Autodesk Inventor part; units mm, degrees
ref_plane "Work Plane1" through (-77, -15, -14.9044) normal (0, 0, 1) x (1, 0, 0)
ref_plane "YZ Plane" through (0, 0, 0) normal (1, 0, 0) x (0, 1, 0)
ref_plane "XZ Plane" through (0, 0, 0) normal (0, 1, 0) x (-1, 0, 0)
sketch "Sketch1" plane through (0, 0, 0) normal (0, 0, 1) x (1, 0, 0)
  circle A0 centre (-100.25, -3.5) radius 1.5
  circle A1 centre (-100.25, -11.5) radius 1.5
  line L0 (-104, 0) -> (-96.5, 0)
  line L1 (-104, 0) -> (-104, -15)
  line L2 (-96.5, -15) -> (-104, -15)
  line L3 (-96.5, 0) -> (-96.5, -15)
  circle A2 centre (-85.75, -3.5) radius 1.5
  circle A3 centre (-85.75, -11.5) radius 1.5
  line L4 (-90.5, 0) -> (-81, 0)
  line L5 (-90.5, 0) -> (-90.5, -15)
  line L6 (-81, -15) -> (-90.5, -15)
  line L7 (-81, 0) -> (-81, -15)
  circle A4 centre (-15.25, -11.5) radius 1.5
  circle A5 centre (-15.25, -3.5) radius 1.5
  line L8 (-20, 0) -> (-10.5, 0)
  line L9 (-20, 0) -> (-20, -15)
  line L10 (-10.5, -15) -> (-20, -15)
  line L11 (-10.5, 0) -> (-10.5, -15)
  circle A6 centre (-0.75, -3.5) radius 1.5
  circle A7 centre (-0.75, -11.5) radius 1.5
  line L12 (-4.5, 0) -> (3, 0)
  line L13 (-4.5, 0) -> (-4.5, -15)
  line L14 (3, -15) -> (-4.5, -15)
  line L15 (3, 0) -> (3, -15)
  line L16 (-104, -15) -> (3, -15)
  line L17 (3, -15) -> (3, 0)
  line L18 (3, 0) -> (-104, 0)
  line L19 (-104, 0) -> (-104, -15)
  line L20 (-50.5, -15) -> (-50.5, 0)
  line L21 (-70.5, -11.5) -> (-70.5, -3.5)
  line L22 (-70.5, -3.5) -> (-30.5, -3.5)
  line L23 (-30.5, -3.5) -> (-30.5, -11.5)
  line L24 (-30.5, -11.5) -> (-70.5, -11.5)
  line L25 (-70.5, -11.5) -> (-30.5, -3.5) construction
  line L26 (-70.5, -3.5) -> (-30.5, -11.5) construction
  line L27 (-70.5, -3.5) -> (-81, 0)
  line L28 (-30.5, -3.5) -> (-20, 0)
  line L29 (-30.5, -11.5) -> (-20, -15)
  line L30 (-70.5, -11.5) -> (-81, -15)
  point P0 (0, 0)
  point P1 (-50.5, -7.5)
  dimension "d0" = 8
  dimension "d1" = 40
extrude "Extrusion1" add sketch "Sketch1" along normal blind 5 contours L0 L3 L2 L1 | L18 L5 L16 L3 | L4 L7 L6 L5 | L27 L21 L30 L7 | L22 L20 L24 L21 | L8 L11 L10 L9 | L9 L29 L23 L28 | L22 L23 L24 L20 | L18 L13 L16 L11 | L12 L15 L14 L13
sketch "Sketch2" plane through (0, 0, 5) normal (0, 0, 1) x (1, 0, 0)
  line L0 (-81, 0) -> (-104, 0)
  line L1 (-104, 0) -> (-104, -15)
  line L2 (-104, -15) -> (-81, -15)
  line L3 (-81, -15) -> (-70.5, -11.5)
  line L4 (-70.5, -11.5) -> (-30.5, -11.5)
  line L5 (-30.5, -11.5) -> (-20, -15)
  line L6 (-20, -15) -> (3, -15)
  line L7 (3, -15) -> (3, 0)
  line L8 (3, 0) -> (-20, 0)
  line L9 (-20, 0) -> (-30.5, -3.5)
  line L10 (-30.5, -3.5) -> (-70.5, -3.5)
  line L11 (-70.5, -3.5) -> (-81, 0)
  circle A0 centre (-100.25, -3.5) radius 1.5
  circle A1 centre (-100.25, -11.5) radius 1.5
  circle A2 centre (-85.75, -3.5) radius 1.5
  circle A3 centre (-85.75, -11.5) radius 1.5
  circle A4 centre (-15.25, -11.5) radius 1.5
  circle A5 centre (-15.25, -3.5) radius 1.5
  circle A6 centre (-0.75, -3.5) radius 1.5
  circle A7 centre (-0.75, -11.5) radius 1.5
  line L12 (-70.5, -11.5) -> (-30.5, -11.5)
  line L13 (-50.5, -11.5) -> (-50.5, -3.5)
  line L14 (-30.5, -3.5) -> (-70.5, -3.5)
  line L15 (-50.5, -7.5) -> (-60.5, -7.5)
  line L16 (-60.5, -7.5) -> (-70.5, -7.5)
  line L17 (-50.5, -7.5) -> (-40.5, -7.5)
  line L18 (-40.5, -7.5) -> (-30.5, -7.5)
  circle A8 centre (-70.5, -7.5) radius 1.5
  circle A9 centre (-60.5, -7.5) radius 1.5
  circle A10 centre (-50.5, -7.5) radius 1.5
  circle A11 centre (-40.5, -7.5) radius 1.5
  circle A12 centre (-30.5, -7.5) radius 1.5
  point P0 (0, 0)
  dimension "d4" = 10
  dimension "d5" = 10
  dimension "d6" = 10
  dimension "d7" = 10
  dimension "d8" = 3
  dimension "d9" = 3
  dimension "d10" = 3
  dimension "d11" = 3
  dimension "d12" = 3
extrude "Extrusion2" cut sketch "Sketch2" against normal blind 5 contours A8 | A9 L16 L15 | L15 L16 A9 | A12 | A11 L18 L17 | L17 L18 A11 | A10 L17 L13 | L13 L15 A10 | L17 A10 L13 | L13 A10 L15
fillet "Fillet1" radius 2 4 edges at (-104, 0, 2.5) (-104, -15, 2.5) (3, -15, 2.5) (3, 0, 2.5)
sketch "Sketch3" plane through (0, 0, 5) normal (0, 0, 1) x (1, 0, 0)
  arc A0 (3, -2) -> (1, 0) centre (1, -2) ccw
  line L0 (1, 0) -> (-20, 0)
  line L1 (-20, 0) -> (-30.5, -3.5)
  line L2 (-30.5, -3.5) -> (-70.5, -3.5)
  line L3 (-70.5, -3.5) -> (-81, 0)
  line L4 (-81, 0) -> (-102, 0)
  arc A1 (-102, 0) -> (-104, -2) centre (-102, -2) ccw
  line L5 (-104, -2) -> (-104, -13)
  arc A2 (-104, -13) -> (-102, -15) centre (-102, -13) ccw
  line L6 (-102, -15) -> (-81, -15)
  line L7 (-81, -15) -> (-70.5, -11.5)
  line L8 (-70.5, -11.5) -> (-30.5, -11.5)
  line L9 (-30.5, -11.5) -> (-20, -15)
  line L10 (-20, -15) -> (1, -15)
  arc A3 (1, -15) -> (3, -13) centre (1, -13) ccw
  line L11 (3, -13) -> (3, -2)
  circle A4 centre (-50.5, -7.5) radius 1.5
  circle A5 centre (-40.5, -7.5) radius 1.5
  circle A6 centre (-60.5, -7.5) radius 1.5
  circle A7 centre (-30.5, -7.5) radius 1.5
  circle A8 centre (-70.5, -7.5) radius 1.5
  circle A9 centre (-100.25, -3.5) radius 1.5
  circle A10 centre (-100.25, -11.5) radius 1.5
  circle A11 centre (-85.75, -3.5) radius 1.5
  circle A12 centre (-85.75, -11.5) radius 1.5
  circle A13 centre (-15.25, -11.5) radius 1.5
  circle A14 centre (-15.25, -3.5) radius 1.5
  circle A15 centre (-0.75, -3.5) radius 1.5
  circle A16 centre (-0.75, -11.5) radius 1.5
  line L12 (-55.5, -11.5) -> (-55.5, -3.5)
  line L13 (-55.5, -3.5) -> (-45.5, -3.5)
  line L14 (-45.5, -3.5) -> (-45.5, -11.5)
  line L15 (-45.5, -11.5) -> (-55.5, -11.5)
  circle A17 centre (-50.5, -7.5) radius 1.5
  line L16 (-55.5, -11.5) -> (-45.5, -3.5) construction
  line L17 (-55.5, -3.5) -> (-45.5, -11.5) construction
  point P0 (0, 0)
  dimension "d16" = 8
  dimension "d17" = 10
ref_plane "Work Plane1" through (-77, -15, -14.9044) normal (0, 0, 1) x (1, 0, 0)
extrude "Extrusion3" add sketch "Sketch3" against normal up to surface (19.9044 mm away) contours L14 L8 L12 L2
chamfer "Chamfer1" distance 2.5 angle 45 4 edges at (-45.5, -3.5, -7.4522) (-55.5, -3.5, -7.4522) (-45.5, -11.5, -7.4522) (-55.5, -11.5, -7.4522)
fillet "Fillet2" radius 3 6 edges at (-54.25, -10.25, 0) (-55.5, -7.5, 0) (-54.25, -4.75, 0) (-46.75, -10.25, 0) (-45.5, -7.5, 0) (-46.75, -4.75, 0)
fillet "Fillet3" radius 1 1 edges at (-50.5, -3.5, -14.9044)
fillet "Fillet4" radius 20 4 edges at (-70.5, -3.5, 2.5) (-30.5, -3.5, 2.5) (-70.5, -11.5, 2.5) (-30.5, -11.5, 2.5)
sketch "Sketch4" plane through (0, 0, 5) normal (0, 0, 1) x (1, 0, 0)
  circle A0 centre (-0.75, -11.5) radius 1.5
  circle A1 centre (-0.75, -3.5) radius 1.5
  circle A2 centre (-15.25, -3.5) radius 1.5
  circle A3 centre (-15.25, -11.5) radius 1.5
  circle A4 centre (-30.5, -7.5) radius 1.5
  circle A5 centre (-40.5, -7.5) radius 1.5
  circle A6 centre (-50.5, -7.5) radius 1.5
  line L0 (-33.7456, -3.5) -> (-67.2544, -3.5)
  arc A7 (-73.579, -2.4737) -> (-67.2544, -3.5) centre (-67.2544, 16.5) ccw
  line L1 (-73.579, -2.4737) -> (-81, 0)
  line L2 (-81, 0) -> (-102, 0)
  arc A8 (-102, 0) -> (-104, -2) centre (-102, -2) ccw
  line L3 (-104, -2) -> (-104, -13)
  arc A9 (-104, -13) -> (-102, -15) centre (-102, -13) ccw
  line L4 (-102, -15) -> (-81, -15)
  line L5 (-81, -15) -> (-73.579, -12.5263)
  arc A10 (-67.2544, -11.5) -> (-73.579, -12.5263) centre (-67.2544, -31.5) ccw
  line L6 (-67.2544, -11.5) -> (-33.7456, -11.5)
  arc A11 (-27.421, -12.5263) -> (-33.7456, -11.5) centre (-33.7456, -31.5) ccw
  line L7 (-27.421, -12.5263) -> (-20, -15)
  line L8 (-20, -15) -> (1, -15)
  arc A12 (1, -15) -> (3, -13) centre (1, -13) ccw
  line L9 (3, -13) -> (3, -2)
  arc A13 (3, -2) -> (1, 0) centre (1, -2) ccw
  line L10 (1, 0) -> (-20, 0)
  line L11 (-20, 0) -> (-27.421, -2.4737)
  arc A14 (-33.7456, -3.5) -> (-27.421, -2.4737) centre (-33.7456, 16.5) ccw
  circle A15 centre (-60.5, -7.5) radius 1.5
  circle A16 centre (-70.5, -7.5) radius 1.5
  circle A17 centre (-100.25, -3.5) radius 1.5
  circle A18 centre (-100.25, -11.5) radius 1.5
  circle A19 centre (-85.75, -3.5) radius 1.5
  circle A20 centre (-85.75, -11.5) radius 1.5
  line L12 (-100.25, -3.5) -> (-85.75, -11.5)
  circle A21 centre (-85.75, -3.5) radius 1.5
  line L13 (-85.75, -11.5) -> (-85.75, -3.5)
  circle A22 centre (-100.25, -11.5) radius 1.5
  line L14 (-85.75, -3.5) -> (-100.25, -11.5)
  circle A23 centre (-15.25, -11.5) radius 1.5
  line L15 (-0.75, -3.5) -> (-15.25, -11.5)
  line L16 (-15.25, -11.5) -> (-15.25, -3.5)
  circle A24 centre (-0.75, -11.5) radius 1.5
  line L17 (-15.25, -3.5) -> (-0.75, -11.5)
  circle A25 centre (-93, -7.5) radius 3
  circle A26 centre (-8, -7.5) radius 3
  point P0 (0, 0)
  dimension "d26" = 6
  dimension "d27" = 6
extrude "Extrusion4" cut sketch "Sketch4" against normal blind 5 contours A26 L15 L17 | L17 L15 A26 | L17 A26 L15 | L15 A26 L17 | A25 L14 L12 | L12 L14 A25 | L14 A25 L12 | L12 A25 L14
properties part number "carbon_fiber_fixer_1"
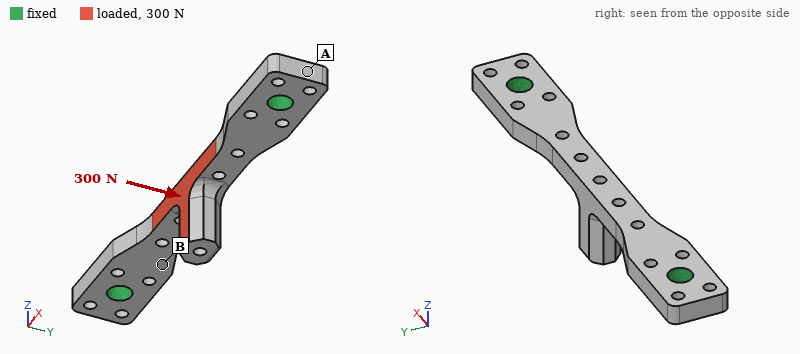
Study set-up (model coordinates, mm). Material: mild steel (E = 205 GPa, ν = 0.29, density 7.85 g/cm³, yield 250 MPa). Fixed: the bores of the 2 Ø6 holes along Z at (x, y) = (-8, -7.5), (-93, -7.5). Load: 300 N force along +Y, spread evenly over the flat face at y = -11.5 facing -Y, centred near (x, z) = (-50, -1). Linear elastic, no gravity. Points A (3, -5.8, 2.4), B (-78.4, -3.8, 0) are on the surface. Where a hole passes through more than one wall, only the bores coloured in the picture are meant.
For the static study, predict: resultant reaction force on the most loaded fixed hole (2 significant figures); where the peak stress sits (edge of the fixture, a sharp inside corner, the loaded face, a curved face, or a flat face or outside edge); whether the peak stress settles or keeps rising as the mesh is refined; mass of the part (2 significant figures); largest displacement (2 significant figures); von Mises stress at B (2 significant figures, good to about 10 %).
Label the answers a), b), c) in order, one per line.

a) 150 N
b) a sharp inside corner
c) keeps rising
d) 51 g
e) 28 µm
f) 13 MPa
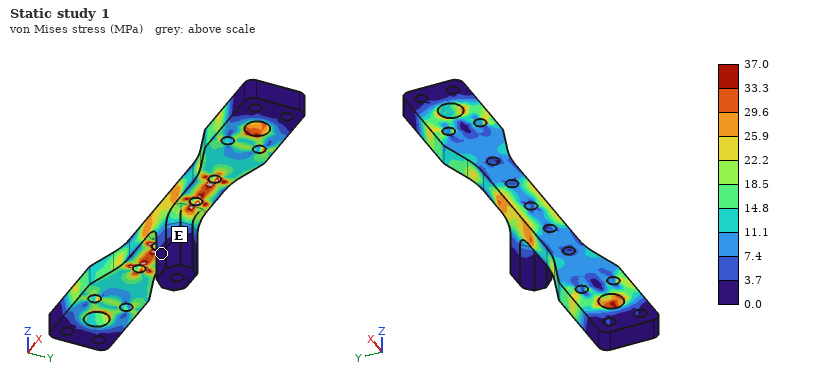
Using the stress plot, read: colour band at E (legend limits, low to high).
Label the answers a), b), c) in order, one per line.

a) 0.0 to 3.7 MPa
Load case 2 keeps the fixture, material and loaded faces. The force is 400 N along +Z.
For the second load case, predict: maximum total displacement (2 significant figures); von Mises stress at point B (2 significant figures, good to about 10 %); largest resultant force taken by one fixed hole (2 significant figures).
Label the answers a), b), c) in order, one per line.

a) 55 µm
b) 31 MPa
c) 210 N
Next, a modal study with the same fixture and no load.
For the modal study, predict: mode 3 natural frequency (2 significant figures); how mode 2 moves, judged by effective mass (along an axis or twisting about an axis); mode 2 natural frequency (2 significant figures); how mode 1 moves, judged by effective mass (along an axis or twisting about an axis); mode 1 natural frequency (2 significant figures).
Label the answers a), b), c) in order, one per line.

a) 7800 Hz
b) along Y
c) 4500 Hz
d) along Z
e) 3500 Hz
